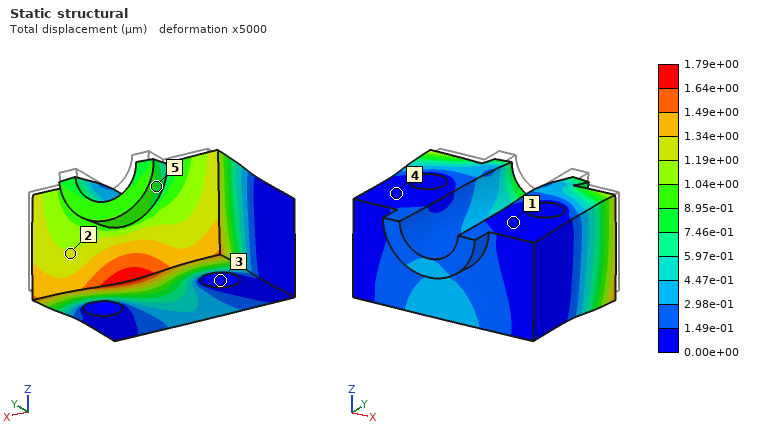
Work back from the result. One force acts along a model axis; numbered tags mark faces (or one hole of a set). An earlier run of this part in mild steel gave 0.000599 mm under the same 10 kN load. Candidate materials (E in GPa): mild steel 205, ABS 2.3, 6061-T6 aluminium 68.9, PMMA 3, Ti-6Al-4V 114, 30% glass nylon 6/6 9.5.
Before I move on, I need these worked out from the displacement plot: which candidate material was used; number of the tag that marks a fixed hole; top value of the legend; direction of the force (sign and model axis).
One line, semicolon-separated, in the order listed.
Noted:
6061-T6 aluminium; 3; 1.79e+00 µm; -Y
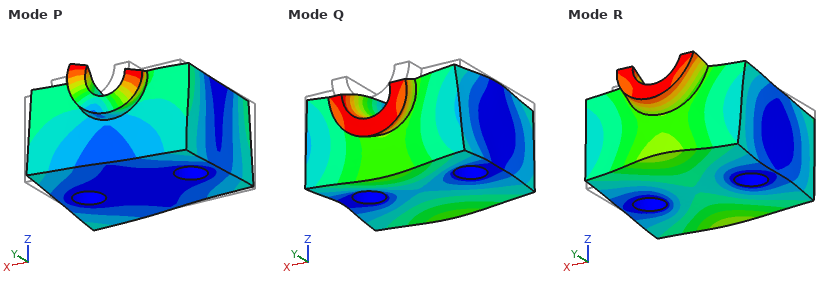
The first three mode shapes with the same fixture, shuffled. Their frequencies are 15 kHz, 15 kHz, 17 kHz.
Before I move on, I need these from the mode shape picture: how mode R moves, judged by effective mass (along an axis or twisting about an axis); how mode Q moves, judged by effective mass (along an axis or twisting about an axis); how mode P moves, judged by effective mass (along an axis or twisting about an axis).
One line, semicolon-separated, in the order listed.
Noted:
twisting about X; along Z; twisting about Z
